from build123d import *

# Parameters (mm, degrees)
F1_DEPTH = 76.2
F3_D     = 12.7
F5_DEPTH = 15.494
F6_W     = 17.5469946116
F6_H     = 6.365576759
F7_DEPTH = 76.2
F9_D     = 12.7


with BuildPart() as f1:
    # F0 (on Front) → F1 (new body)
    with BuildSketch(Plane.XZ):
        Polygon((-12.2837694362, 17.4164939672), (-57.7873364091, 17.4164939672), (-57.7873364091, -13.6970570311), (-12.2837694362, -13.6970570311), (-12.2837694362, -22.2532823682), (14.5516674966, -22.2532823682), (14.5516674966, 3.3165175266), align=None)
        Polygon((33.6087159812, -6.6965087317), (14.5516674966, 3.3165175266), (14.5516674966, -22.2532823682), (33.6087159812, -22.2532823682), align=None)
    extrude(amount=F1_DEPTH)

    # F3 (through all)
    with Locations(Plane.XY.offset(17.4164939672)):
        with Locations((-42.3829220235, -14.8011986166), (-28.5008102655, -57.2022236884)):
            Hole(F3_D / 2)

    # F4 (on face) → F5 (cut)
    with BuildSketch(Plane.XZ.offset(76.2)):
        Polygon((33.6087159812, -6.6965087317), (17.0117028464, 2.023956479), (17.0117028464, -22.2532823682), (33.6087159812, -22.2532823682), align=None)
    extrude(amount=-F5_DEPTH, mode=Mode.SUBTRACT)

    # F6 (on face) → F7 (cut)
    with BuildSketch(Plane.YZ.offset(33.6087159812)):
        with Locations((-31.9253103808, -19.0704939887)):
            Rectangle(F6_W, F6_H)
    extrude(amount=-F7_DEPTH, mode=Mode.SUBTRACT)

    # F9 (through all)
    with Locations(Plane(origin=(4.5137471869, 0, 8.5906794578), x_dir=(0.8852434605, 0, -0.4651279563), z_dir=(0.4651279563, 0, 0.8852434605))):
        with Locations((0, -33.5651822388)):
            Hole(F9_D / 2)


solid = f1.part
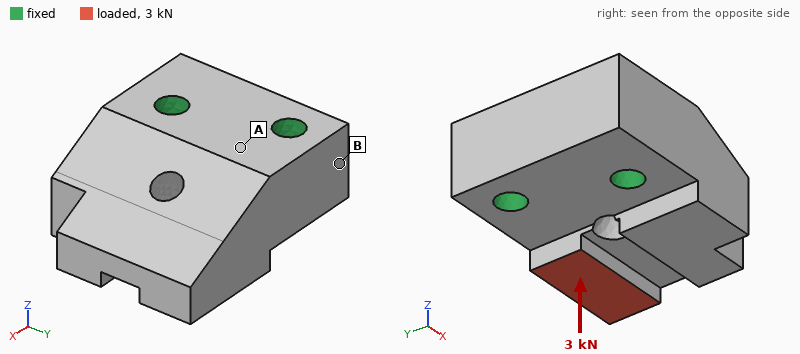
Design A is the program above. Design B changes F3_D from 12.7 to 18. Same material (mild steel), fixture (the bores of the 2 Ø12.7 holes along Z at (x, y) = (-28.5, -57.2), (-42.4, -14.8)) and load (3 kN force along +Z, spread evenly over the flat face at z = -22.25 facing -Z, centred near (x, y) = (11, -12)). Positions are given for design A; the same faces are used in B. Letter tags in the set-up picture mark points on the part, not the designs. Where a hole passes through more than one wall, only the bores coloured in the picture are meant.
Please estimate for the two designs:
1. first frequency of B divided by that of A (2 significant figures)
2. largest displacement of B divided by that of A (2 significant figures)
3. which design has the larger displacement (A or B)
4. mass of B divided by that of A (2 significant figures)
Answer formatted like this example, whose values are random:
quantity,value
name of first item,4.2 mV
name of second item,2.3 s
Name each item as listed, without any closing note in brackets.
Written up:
quantity,value
first frequency of B divided by that of A,1.1
largest displacement of B divided by that of A,0.89
which design has the larger displacement,A
mass of B divided by that of A,0.96
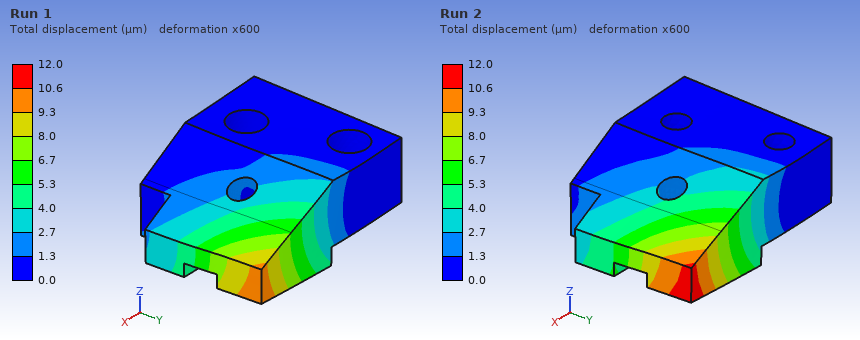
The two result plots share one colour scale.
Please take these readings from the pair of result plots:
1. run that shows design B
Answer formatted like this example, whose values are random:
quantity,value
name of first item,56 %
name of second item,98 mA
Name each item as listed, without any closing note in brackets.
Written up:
quantity,value
run that shows design B,Run 1
